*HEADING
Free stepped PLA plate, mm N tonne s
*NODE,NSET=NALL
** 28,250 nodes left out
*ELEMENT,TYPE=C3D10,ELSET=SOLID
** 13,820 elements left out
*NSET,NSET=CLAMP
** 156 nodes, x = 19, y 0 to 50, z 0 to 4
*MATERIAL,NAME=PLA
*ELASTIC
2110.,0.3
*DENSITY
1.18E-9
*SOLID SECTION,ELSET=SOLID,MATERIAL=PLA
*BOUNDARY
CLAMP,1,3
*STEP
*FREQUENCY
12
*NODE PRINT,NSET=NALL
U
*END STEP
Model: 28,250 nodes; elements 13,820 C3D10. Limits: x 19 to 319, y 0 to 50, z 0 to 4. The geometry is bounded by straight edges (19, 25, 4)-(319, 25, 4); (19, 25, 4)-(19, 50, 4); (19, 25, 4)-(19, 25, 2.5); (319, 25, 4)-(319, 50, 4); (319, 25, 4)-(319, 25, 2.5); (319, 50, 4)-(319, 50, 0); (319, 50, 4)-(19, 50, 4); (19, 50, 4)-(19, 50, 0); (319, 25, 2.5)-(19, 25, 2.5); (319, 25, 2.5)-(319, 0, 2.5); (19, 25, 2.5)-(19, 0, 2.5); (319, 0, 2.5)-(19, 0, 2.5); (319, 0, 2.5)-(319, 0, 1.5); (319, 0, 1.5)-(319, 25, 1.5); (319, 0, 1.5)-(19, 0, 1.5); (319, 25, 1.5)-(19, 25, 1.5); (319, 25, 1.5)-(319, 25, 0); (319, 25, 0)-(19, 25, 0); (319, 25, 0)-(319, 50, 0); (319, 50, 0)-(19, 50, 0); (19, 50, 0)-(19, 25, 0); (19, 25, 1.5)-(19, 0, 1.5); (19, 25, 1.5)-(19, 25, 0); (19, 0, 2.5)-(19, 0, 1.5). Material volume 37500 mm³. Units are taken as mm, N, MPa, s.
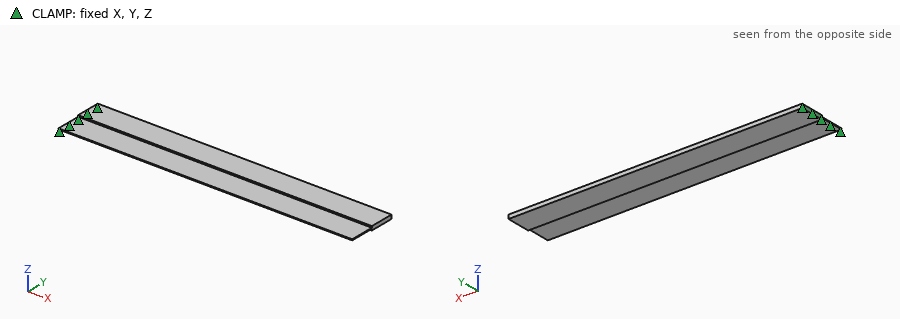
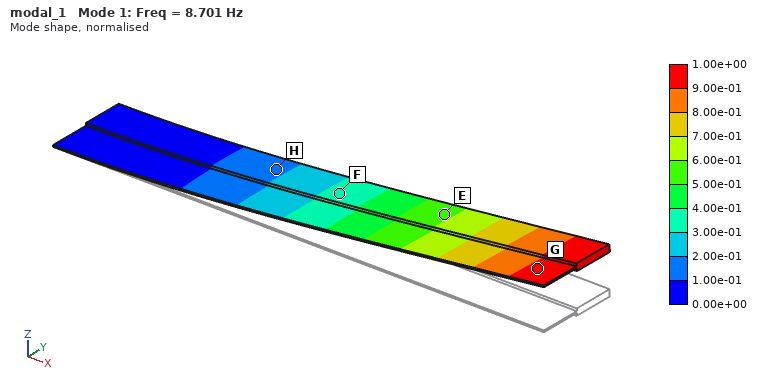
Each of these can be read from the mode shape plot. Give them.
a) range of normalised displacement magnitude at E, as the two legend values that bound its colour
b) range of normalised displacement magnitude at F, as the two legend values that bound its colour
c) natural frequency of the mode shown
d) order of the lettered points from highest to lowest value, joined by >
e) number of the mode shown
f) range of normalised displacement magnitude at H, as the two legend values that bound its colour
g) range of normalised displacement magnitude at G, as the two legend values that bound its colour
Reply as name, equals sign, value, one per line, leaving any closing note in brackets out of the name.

range of normalised displacement magnitude at E, as the two legend values that bound its colour = 5.00e-01 to 6.00e-01
range of normalised displacement magnitude at F, as the two legend values that bound its colour = 3.00e-01 to 4.00e-01
natural frequency of the mode shown = 8.701 Hz
order of the lettered points from highest to lowest value, joined by > = G > E > F > H
number of the mode shown = 1
range of normalised displacement magnitude at H, as the two legend values that bound its colour = 1.00e-01 to 2.00e-01
range of normalised displacement magnitude at G, as the two legend values that bound its colour = 9.00e-01 to 1.00e+00
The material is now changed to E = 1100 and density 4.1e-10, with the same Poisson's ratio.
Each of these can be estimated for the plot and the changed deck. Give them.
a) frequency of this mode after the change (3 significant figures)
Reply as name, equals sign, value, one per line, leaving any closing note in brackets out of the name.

frequency of this mode after the change = 10.7 Hz
